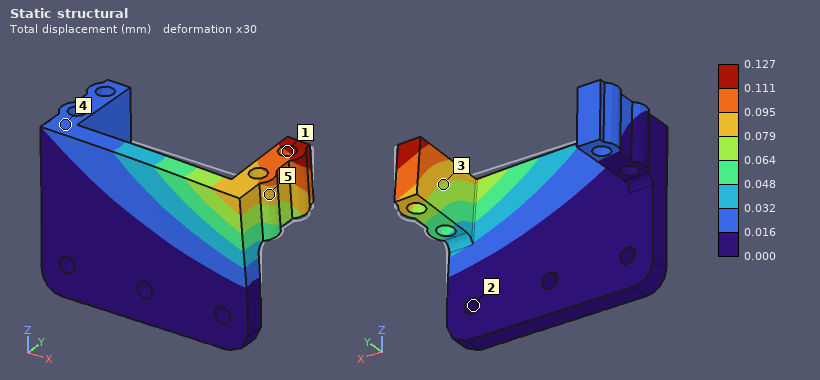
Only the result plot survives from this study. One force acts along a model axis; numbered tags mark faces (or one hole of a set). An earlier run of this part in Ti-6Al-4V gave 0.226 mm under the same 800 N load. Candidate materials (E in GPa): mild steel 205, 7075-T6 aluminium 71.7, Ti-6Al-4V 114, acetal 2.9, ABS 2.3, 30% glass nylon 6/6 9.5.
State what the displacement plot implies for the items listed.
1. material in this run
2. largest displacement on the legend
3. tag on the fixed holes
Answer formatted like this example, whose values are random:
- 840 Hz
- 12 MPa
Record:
- mild steel
- 0.127 mm
- 2
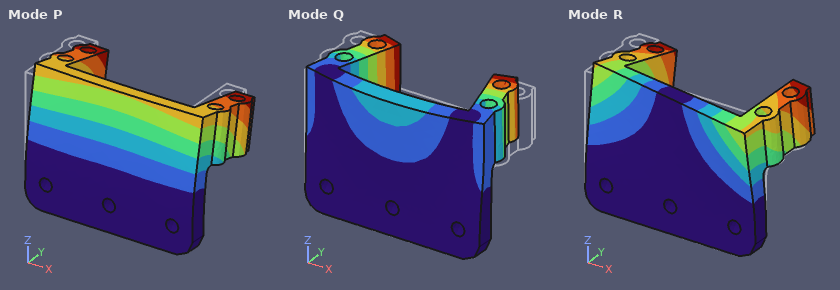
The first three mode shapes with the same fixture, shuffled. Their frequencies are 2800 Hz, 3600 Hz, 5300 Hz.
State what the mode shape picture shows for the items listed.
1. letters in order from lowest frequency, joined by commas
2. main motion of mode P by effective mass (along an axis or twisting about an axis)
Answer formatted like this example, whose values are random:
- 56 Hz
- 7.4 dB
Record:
- P, R, Q
- along Y
